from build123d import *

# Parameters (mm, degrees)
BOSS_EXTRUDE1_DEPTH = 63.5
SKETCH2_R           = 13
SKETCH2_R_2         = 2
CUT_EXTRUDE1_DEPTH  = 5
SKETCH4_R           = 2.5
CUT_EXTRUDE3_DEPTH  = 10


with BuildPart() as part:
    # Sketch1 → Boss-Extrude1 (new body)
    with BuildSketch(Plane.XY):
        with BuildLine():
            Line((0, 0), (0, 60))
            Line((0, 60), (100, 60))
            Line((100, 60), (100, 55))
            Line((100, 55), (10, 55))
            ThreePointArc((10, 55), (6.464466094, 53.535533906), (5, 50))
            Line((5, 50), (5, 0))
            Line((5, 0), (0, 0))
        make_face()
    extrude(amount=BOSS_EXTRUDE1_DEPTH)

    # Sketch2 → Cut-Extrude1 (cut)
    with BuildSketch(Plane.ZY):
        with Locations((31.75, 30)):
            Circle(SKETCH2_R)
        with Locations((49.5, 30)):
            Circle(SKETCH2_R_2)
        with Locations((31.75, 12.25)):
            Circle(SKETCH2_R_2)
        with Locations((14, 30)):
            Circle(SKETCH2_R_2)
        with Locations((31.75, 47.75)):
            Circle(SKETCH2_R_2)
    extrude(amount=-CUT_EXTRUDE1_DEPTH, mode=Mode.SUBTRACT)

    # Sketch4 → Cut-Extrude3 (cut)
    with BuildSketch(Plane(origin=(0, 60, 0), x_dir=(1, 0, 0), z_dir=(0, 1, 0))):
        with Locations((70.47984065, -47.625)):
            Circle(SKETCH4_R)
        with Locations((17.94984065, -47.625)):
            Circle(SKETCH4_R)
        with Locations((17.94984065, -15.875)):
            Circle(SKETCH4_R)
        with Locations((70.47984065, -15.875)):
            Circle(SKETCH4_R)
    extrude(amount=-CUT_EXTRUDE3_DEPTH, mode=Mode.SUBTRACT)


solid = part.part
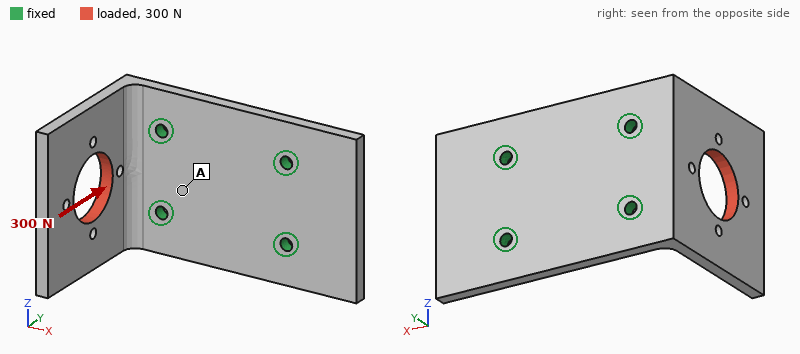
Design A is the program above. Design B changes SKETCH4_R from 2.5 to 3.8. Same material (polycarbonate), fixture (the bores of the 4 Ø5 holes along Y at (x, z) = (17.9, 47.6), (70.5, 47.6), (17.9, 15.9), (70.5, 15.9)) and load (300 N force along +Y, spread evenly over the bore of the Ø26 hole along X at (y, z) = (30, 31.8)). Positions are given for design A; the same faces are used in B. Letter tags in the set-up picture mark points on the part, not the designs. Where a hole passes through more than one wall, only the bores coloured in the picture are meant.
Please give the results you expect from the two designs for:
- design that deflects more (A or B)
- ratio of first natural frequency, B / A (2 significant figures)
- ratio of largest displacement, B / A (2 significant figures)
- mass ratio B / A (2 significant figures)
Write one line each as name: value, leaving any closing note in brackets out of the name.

design that deflects more: A
ratio of first natural frequency, B / A: 1.0
ratio of largest displacement, B / A: 0.77
mass ratio B / A: 0.99
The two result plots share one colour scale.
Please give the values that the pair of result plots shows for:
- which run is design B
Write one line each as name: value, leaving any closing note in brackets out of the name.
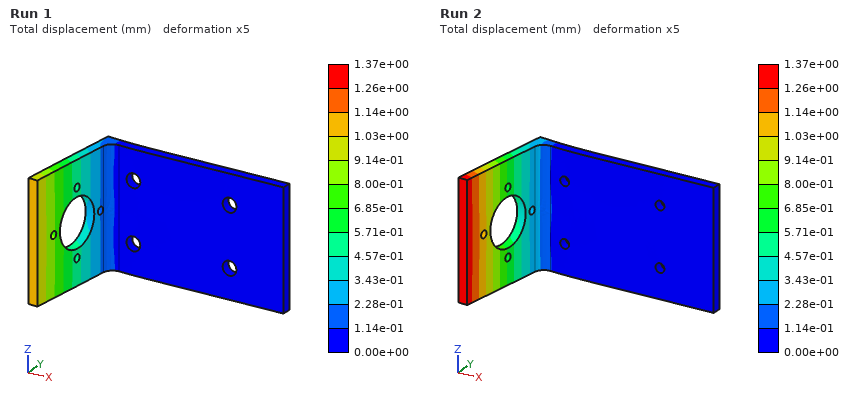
which run is design B: Run 1
